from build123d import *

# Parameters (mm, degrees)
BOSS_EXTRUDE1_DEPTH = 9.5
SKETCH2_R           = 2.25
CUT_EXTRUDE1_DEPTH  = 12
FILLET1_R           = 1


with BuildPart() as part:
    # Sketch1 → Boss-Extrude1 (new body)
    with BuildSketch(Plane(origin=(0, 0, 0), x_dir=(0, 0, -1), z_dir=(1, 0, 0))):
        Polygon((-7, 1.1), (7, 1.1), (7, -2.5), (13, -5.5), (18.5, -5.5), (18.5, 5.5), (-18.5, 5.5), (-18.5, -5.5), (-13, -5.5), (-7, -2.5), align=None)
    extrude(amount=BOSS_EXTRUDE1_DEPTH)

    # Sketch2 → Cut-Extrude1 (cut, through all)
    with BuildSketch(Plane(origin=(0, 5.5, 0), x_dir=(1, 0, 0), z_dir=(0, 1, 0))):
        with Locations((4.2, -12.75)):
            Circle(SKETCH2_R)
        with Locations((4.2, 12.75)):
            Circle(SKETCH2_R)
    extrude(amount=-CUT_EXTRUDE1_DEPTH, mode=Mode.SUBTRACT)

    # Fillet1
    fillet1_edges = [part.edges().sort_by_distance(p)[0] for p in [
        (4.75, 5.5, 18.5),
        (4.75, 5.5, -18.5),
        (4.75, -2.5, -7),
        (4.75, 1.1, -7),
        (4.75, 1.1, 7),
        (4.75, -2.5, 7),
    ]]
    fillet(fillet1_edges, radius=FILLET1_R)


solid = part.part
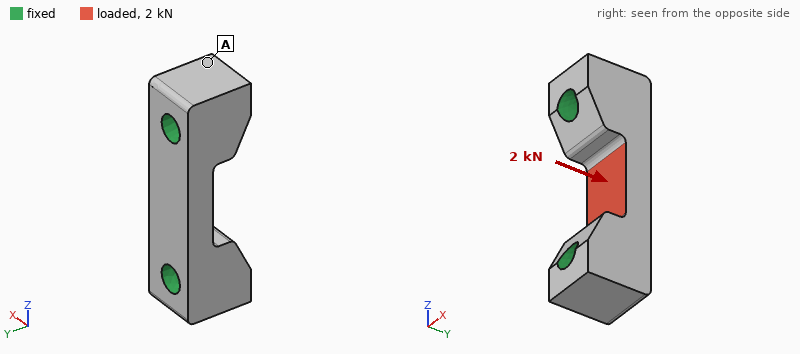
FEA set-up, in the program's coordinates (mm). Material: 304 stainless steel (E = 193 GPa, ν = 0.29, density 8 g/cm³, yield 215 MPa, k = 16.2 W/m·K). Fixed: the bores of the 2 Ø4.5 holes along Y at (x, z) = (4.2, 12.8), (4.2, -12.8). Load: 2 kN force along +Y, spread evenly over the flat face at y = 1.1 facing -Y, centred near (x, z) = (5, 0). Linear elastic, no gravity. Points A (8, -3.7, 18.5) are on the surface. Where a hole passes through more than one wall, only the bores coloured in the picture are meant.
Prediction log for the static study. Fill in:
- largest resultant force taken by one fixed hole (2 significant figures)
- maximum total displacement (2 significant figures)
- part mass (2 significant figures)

1.0 kN
5.8 µm
20 g
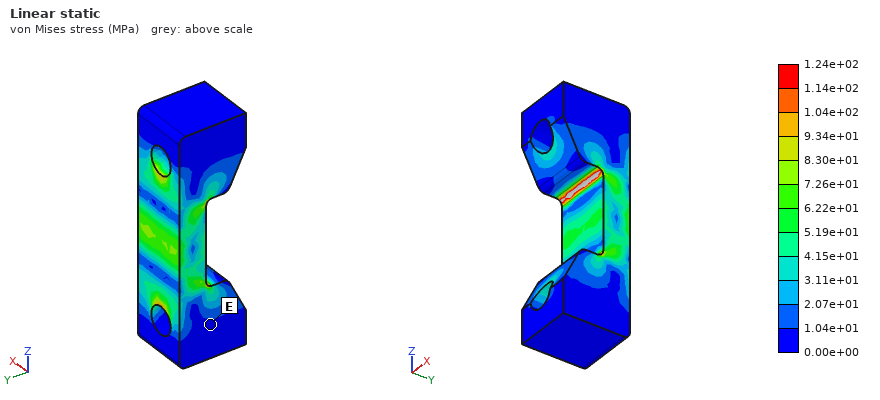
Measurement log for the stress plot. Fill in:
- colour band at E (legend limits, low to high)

0.00e+00 to 1.04e+01 MPa
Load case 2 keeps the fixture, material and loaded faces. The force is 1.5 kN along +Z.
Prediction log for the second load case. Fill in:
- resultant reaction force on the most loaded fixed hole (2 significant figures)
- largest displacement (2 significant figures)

770 N
1.2 µm
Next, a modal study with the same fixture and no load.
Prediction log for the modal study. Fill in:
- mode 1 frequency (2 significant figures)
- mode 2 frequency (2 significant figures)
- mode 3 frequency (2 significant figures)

51 kHz
52 kHz
69 kHz
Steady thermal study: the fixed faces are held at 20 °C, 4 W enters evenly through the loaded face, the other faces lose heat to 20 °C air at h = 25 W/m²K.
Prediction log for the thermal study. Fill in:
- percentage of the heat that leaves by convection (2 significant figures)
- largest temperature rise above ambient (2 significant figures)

3.5 %
23 K
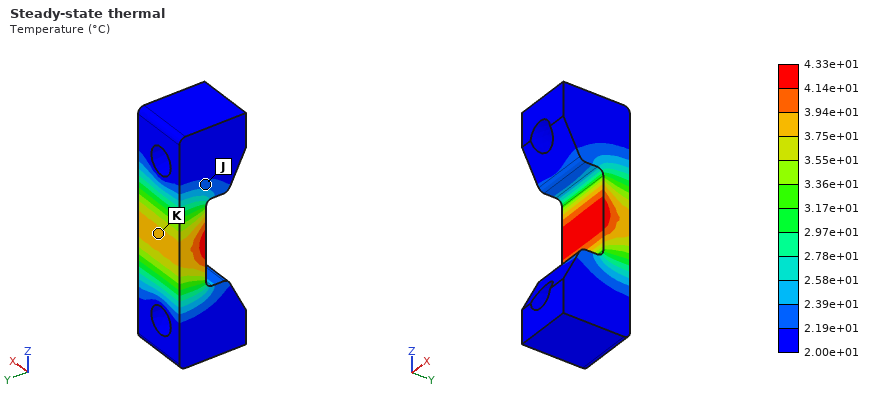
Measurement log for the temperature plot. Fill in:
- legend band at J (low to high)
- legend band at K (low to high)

2.19e+01 to 2.39e+01 °C
3.75e+01 to 3.94e+01 °C
